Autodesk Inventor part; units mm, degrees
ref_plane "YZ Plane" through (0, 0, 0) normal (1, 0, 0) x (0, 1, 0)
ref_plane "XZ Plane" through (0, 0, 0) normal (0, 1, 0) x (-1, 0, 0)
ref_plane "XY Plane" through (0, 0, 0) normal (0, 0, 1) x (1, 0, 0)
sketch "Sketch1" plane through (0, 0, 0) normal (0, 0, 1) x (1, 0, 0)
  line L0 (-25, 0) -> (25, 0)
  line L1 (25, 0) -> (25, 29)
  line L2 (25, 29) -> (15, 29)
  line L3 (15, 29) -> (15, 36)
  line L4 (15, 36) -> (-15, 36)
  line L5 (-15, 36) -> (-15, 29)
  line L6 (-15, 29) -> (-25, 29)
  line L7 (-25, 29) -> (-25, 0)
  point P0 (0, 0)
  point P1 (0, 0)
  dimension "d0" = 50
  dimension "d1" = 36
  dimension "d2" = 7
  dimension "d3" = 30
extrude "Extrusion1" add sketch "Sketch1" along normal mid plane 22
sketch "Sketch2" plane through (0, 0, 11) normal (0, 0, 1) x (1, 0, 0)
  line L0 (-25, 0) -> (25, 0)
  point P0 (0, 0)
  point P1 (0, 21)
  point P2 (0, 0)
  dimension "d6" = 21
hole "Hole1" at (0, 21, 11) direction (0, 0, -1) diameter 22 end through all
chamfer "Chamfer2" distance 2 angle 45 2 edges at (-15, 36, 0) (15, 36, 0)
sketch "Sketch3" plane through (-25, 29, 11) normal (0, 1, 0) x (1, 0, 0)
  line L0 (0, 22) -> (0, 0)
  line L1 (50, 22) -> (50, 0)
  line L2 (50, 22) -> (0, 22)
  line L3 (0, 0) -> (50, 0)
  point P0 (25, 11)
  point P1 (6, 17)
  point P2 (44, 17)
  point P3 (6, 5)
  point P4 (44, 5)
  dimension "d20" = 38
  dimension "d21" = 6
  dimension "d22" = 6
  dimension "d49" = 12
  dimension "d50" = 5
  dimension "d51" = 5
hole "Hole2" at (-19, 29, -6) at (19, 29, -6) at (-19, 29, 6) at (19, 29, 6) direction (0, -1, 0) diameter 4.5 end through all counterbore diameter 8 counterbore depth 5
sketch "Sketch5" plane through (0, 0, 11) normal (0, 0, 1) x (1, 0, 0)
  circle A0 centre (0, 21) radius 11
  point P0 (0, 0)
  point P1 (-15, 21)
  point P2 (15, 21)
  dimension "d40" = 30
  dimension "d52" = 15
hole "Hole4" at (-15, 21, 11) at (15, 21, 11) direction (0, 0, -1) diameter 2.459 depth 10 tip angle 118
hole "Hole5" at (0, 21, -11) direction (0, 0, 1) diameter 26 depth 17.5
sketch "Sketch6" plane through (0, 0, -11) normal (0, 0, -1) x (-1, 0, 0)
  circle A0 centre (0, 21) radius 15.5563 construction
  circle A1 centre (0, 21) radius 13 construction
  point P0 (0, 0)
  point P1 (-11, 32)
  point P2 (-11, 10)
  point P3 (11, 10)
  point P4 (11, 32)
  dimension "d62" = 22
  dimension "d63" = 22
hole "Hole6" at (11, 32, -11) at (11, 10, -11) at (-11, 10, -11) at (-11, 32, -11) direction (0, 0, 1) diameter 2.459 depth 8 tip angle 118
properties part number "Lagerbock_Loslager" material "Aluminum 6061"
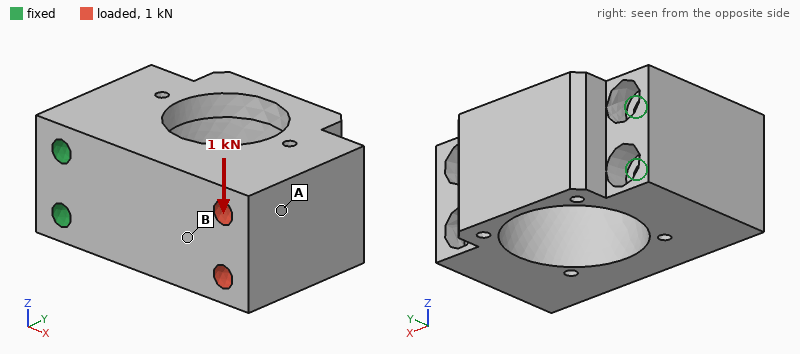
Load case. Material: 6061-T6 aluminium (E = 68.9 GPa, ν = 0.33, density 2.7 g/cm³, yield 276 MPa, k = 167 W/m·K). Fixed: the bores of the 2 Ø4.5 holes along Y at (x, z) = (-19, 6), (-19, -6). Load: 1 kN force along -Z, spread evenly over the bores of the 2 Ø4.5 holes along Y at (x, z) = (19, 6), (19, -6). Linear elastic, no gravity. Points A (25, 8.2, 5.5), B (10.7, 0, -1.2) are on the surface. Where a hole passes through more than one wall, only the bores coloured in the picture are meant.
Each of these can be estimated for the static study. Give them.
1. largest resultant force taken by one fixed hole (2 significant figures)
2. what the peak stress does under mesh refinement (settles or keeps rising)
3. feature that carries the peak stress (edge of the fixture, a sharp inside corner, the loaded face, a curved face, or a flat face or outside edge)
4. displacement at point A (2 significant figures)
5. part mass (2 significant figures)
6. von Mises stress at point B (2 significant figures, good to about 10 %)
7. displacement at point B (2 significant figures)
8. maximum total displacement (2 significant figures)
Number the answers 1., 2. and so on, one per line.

1. 2.6 kN
2. keeps rising
3. edge of the fixture
4. 37 µm
5. 61 g
6. 10 MPa
7. 19 µm
8. 44 µm
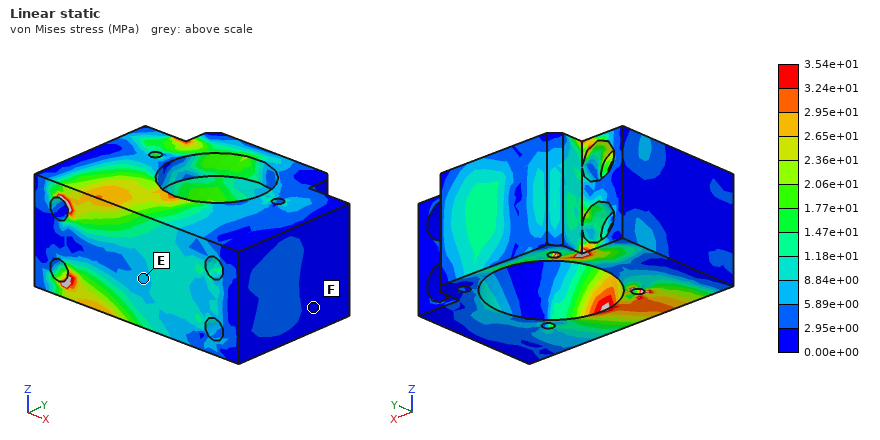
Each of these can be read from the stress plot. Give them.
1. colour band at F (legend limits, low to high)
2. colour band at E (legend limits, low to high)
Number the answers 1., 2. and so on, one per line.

1. 0.00e+00 to 2.95e+00 MPa
2. 5.89e+00 to 8.84e+00 MPa
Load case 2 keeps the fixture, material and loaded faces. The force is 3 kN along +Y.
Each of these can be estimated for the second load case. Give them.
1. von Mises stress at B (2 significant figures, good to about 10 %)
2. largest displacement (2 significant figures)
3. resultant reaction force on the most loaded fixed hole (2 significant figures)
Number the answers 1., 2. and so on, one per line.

1. 12 MPa
2. 0.16 mm
3. 1.6 kN
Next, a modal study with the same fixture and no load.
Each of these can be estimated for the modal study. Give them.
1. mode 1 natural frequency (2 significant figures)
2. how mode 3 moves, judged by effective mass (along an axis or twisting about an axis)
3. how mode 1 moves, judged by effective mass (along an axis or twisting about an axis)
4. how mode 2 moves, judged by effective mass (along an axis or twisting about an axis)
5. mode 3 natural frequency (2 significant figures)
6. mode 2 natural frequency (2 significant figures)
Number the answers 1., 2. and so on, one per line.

1. 4600 Hz
2. twisting about X
3. along Y
4. along Z
5. 11 kHz
6. 5600 Hz
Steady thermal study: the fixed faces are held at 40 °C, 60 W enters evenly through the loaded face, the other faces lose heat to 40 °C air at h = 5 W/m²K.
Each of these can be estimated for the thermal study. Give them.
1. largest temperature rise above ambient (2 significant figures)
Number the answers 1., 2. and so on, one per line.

1. 44 K
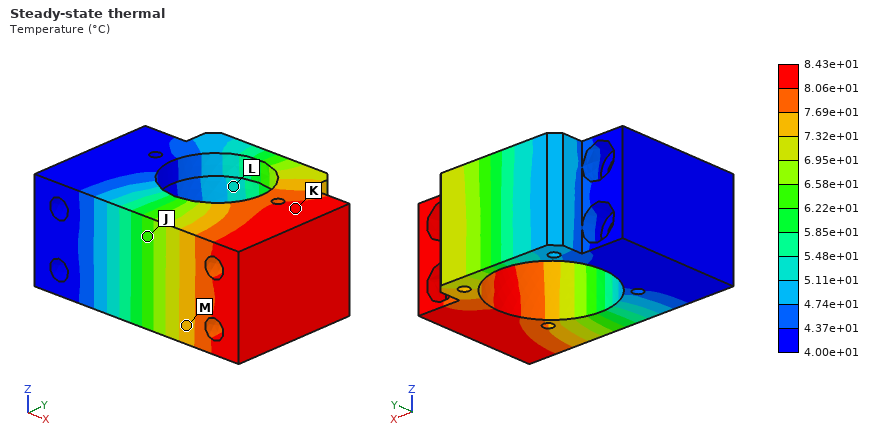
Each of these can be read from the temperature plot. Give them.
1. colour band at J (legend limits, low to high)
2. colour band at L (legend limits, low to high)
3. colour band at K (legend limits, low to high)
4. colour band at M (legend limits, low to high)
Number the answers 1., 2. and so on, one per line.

1. 6.22e+01 to 6.58e+01 °C
2. 5.11e+01 to 5.48e+01 °C
3. 8.06e+01 to 8.43e+01 °C
4. 7.32e+01 to 7.69e+01 °C
